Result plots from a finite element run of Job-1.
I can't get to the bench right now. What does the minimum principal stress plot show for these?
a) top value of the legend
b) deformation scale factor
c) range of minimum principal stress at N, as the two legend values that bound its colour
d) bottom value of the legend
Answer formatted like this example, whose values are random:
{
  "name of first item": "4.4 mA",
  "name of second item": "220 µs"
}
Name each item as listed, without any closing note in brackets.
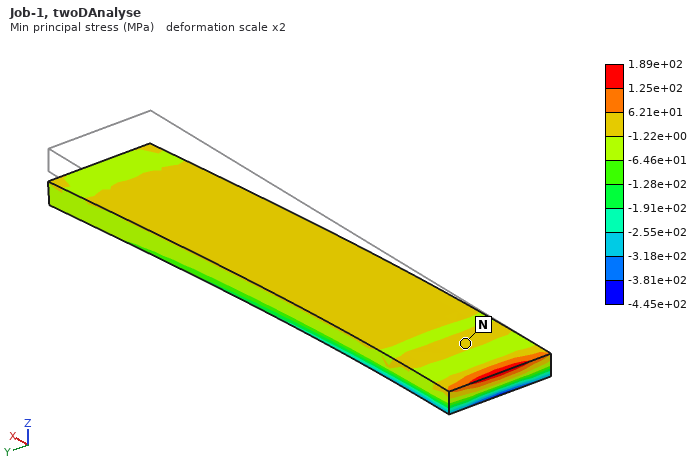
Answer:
{
  "top value of the legend": "1.89e+02 MPa",
  "deformation scale factor": "2",
  "range of minimum principal stress at N, as the two legend values that bound its colour": "-1.22e+00 to 6.21e+01 MPa",
  "bottom value of the legend": "-4.45e+02 MPa"
}
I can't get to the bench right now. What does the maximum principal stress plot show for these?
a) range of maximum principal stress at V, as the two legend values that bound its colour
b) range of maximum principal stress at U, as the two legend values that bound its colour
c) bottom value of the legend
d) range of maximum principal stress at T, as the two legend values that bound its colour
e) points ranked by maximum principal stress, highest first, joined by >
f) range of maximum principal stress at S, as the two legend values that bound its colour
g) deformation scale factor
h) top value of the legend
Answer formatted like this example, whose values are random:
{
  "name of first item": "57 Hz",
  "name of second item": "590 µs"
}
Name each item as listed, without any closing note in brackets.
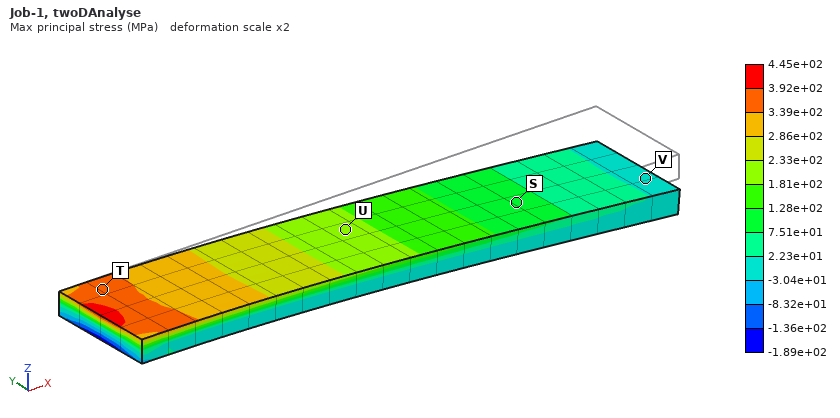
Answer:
{
  "range of maximum principal stress at V, as the two legend values that bound its colour": "-3.04e+01 to 2.23e+01 MPa",
  "range of maximum principal stress at U, as the two legend values that bound its colour": "1.81e+02 to 2.33e+02 MPa",
  "bottom value of the legend": "-1.89e+02 MPa",
  "range of maximum principal stress at T, as the two legend values that bound its colour": "3.39e+02 to 3.92e+02 MPa",
  "points ranked by maximum principal stress, highest first, joined by >": "T > U > S > V",
  "range of maximum principal stress at S, as the two legend values that bound its colour": "7.51e+01 to 1.28e+02 MPa",
  "deformation scale factor": "2",
  "top value of the legend": "4.45e+02 MPa"
}
